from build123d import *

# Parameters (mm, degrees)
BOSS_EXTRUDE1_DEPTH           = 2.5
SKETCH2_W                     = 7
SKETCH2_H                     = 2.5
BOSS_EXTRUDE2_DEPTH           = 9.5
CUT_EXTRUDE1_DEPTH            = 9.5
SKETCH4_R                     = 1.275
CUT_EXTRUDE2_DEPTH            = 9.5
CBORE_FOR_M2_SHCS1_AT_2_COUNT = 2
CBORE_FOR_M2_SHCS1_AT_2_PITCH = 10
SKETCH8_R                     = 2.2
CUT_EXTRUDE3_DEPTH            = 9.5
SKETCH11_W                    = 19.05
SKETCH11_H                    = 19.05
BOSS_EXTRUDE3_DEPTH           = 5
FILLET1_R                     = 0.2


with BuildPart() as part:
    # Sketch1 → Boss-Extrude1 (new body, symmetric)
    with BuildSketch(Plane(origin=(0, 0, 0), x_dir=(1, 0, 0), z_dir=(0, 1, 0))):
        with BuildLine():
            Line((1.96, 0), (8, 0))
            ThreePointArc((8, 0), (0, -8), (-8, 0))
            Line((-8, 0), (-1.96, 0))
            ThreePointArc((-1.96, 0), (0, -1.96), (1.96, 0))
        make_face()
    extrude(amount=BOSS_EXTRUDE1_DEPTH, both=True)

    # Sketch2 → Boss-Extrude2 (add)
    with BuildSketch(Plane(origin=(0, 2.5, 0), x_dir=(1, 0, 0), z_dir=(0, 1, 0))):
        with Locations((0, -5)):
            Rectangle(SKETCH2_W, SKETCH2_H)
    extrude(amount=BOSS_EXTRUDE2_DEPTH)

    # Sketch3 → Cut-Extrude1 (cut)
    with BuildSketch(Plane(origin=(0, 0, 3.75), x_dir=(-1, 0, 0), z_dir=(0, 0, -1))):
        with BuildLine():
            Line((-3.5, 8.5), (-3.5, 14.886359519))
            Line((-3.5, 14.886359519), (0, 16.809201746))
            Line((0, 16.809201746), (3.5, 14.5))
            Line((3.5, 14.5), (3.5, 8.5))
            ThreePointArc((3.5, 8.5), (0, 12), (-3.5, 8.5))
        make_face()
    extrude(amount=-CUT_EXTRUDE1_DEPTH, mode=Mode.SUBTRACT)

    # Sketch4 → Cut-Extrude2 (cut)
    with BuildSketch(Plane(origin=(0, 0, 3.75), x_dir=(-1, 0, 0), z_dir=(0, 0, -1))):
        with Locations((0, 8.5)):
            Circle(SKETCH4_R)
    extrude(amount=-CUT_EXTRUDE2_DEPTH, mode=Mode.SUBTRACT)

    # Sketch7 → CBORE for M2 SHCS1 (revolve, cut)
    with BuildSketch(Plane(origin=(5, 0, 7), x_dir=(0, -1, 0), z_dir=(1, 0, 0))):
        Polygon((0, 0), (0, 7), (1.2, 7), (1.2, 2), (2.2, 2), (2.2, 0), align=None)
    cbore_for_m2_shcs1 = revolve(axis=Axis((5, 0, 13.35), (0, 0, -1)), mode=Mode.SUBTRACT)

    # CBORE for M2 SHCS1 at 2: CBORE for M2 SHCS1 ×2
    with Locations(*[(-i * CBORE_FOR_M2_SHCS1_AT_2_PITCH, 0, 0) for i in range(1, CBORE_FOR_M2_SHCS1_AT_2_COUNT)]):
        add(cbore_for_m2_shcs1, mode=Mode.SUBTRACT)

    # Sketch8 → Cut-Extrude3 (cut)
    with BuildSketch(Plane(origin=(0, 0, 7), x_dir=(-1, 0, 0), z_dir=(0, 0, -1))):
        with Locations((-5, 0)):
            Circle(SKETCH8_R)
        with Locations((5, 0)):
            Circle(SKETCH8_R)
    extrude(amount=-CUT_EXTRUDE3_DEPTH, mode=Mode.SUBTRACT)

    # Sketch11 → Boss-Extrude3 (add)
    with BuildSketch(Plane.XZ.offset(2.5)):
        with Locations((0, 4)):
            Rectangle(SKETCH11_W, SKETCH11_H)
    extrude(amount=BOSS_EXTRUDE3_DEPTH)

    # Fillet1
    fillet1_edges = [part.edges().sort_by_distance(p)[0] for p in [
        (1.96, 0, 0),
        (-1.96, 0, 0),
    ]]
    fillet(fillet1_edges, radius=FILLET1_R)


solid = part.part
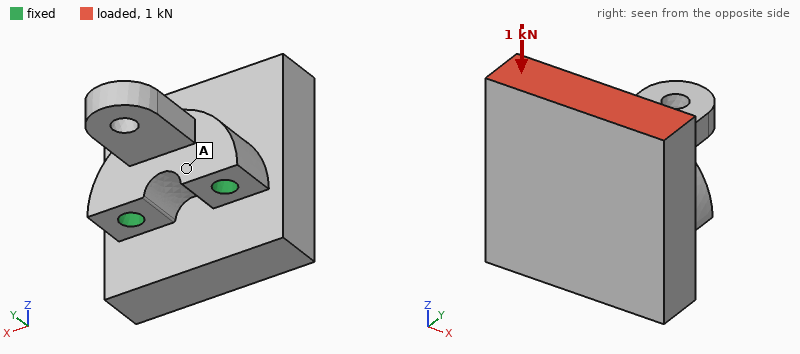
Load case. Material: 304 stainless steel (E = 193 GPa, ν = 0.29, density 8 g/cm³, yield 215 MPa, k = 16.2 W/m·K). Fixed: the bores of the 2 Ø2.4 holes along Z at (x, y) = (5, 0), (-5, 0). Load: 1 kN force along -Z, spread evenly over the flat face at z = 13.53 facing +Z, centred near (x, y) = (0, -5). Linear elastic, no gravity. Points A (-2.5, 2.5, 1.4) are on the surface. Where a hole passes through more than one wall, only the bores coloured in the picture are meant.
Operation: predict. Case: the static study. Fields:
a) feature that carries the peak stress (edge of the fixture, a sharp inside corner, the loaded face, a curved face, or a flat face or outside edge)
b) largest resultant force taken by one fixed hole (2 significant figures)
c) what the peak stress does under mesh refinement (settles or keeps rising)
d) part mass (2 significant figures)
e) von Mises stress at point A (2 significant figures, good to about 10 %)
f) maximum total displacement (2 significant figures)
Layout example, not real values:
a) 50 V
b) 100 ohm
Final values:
a) edge of the fixture
b) 500 N
c) keeps rising
d) 19 g
e) 16 MPa
f) 5.8 µm
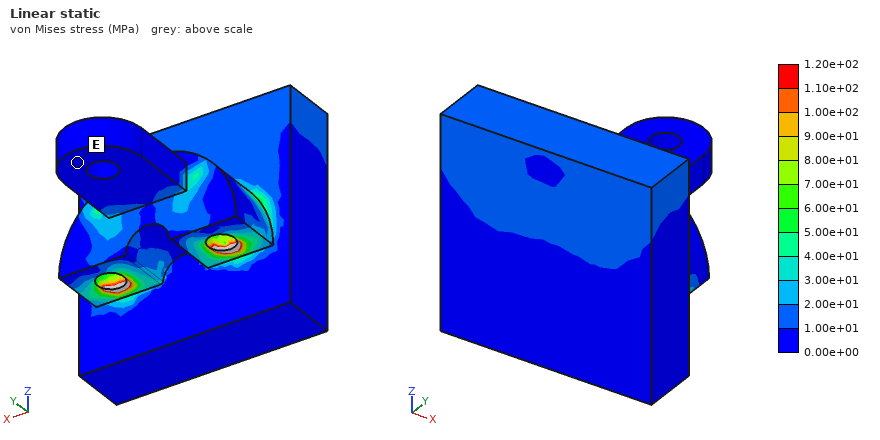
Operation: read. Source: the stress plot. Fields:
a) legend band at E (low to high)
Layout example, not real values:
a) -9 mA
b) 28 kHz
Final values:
a) 0.00e+00 to 1.00e+01 MPa
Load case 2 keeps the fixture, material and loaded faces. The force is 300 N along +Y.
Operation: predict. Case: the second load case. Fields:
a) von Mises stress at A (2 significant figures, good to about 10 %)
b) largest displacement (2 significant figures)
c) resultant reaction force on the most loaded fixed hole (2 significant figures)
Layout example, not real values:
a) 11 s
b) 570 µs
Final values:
a) 16 MPa
b) 6.4 µm
c) 160 N
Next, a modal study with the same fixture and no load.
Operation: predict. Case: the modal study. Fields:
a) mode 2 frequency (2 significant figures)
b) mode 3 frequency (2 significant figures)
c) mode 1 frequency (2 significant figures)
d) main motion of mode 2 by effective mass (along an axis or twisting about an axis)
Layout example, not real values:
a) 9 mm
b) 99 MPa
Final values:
a) 22 kHz
b) 29 kHz
c) 17 kHz
d) along Z
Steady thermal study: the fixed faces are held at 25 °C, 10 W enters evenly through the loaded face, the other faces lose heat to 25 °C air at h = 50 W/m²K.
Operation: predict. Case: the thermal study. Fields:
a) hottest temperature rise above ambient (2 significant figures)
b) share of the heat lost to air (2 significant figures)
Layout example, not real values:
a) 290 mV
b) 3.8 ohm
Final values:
a) 79 K
b) 18 %
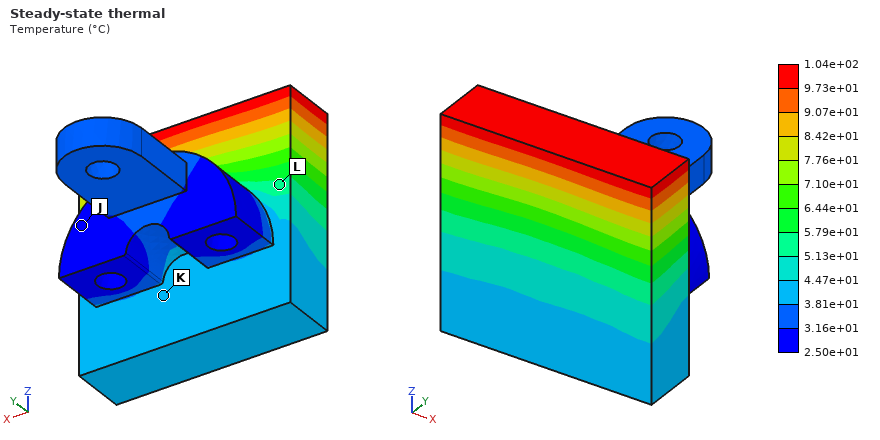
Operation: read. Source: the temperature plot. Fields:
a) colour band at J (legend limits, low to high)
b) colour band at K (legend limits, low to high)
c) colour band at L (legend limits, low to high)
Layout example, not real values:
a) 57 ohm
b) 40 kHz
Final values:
a) 2.50e+01 to 3.16e+01 °C
b) 3.81e+01 to 4.47e+01 °C
c) 5.13e+01 to 5.79e+01 °C
